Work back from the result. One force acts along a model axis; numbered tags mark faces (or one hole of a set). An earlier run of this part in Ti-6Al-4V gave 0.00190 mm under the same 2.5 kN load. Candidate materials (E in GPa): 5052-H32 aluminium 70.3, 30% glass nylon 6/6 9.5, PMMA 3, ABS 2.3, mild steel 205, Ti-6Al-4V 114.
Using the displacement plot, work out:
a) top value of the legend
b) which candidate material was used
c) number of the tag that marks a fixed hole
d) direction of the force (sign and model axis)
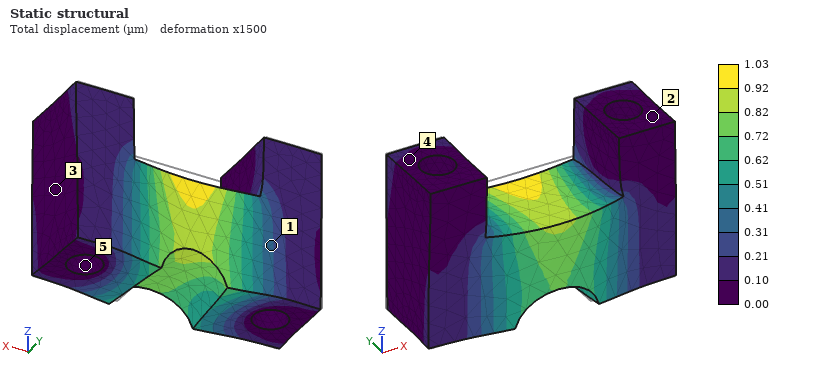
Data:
1.03 µm
mild steel
5
-Y
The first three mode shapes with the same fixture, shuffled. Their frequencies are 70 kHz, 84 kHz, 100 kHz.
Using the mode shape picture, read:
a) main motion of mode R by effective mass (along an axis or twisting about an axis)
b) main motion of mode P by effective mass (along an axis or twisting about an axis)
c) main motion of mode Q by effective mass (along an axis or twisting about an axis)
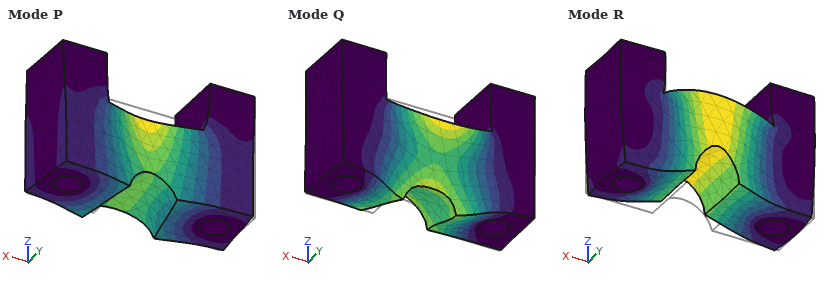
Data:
along Z
along Y
twisting about X
